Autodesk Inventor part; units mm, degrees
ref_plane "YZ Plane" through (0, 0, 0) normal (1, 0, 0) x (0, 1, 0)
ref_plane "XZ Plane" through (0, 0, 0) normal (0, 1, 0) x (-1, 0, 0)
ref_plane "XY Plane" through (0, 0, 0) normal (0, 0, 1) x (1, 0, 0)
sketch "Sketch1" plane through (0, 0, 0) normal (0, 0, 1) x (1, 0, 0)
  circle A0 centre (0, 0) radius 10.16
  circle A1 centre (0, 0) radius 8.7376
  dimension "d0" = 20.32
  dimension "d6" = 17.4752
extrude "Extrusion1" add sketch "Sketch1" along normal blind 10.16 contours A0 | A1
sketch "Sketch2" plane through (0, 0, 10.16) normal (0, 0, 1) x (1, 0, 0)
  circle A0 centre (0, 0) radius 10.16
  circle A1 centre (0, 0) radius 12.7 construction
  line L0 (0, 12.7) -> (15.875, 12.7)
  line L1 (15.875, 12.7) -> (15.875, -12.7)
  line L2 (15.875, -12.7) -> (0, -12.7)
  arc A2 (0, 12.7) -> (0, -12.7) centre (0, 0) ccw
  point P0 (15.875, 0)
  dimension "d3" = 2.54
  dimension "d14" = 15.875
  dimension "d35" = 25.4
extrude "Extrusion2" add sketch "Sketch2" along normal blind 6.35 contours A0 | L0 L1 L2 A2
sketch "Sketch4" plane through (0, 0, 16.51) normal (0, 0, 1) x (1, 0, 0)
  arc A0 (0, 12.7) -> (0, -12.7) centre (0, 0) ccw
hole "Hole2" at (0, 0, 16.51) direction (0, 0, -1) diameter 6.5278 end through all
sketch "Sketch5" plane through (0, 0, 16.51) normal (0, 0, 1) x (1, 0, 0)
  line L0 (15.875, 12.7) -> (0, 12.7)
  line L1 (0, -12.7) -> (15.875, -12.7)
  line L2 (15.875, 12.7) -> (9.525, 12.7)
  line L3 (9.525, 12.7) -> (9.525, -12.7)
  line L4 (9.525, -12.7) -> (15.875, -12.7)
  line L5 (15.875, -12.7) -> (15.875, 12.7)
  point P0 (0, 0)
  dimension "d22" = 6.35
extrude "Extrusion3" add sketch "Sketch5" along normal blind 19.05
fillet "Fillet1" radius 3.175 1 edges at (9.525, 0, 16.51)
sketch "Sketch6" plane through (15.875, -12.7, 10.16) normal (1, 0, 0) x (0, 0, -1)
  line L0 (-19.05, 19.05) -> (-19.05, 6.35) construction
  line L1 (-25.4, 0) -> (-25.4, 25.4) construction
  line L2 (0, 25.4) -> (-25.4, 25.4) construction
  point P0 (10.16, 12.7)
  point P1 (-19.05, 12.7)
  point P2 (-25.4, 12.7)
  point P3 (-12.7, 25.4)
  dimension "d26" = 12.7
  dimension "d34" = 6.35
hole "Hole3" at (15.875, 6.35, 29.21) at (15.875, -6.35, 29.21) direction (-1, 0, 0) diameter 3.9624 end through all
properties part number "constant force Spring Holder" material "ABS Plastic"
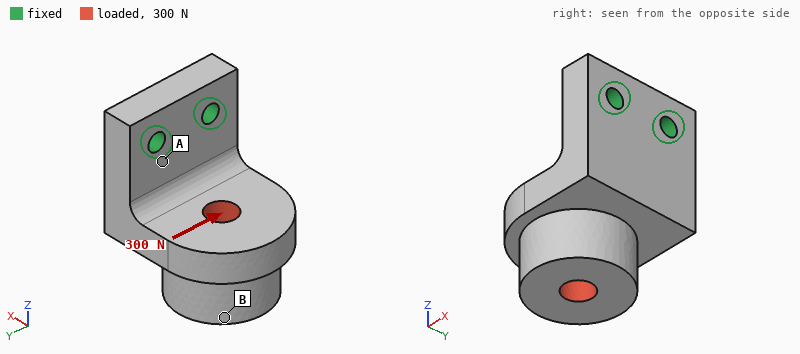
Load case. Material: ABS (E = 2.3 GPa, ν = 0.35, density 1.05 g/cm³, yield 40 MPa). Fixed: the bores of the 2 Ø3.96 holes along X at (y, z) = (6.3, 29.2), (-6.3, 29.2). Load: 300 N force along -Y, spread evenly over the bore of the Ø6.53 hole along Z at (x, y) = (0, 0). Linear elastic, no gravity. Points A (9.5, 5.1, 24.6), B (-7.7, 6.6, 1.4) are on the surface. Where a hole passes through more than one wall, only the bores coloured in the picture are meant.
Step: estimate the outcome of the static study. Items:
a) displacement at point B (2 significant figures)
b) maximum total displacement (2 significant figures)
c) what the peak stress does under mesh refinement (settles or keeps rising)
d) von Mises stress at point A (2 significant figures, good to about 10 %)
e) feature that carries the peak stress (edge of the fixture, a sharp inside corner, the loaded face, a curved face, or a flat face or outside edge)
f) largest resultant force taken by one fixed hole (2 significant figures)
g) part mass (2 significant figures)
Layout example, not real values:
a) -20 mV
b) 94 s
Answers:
a) 0.44 mm
b) 0.49 mm
c) keeps rising
d) 14 MPa
e) edge of the fixture
f) 470 N
g) 10 g
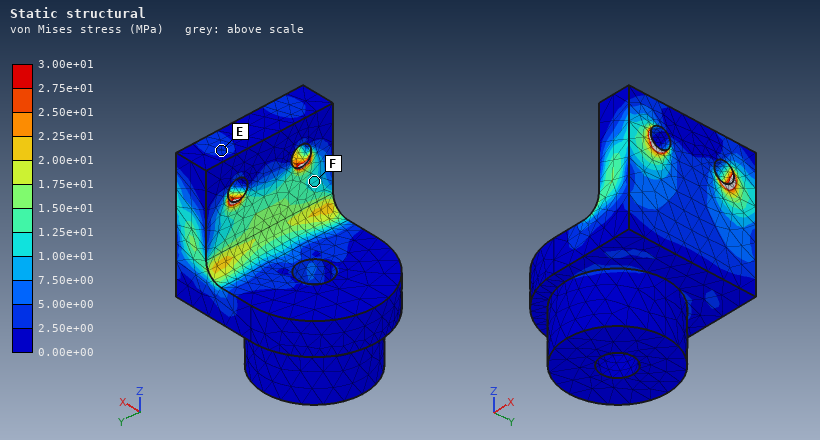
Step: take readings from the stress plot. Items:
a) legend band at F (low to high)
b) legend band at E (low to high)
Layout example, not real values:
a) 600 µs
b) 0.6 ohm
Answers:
a) 1.00e+01 to 1.25e+01 MPa
b) 2.50e+00 to 5.00e+00 MPa
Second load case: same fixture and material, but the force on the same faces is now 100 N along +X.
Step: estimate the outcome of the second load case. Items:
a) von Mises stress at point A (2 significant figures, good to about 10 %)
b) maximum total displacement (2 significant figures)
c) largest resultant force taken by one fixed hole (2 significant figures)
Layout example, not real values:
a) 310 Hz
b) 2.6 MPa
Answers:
a) 10 MPa
b) 0.53 mm
c) 50 N
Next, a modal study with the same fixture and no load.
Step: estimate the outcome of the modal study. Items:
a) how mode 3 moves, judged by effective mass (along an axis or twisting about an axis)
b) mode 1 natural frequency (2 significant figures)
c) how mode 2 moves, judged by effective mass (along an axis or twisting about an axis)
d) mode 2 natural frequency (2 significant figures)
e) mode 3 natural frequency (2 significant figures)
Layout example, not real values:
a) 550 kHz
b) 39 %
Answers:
a) along X
b) 920 Hz
c) along Y
d) 1800 Hz
e) 3800 Hz
